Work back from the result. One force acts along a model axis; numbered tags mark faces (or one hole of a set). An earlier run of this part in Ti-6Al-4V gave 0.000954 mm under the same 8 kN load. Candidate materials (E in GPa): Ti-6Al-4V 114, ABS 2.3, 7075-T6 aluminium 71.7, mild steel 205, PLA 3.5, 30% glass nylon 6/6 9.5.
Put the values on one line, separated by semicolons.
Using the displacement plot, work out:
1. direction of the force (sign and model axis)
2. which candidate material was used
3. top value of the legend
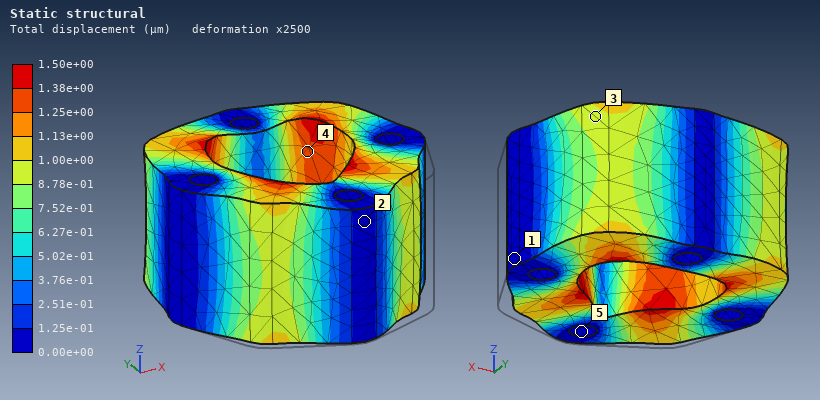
+Y; 7075-T6 aluminium; 1.50e+00 µm
